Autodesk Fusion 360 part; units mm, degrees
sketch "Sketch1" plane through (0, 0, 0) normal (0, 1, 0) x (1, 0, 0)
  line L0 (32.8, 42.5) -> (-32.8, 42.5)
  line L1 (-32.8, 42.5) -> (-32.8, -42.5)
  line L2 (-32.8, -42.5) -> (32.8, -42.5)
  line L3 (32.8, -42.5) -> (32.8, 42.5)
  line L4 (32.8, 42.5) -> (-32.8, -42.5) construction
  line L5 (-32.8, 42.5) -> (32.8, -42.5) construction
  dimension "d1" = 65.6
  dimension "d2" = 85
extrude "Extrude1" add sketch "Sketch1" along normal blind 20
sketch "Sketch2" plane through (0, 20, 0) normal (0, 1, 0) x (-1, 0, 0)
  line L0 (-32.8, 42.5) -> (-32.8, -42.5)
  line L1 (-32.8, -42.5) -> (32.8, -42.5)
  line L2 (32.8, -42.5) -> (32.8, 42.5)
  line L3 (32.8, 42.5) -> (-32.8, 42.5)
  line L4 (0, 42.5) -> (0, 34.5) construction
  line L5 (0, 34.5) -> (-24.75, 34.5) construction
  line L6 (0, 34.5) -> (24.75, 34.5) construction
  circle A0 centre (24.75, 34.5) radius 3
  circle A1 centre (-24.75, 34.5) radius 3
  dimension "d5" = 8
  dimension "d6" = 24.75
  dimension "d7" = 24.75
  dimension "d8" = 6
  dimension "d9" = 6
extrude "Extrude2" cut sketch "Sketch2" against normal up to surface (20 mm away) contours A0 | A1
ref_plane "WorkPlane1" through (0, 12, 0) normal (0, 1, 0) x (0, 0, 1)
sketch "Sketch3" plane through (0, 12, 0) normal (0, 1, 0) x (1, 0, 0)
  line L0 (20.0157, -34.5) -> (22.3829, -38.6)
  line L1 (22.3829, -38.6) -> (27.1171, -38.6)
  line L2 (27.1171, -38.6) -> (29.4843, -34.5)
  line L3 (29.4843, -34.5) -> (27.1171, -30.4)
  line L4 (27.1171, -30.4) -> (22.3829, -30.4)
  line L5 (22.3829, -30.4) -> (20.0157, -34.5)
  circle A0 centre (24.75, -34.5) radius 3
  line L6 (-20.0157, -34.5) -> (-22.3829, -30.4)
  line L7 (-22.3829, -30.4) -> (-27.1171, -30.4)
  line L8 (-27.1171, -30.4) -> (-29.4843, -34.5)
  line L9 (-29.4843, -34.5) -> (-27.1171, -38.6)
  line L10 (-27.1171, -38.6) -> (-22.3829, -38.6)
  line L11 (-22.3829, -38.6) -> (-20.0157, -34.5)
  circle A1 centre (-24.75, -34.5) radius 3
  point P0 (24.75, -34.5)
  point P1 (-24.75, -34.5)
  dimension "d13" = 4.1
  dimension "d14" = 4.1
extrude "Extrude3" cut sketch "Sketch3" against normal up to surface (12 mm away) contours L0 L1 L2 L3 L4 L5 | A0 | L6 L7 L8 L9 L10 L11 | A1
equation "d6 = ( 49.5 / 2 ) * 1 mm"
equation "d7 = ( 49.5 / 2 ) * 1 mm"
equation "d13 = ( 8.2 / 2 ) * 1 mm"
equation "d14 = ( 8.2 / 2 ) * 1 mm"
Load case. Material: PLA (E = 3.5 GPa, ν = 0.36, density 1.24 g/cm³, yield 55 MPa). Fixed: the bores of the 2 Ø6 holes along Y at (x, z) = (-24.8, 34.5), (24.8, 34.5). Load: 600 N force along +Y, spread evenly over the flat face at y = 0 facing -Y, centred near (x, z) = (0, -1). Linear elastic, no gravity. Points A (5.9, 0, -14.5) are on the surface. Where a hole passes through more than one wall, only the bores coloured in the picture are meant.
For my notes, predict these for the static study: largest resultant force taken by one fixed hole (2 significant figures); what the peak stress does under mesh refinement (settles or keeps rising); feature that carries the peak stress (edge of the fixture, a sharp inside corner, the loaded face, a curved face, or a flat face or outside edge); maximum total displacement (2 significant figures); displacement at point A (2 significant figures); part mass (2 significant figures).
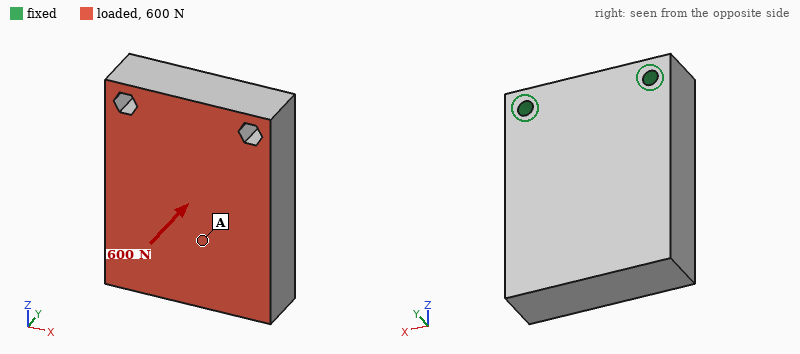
310 N
keeps rising
edge of the fixture
0.96 mm
0.61 mm
140 g
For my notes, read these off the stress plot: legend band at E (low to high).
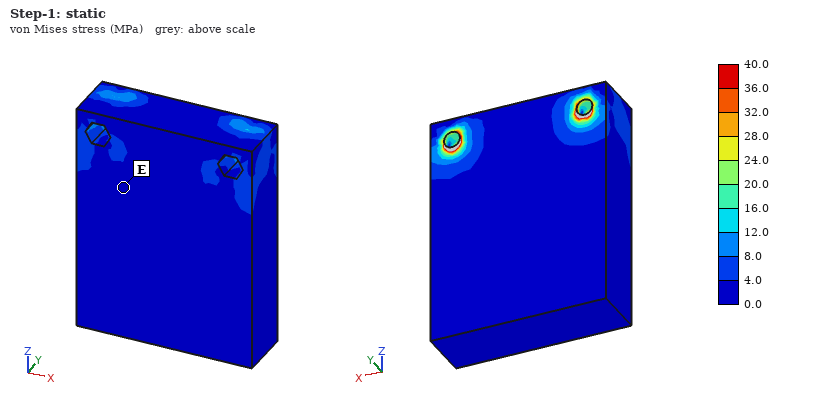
0.0 to 4.0 MPa
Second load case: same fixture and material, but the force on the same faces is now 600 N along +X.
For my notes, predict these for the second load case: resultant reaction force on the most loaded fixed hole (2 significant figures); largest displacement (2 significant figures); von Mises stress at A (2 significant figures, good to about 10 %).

540 N
67 µm
0.88 MPa
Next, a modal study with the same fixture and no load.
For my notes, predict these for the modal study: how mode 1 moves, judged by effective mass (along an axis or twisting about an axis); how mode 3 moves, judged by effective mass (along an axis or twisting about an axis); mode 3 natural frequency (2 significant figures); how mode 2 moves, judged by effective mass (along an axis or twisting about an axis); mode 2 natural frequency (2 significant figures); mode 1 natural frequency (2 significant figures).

along Y
along X
1900 Hz
along X
1600 Hz
420 Hz
